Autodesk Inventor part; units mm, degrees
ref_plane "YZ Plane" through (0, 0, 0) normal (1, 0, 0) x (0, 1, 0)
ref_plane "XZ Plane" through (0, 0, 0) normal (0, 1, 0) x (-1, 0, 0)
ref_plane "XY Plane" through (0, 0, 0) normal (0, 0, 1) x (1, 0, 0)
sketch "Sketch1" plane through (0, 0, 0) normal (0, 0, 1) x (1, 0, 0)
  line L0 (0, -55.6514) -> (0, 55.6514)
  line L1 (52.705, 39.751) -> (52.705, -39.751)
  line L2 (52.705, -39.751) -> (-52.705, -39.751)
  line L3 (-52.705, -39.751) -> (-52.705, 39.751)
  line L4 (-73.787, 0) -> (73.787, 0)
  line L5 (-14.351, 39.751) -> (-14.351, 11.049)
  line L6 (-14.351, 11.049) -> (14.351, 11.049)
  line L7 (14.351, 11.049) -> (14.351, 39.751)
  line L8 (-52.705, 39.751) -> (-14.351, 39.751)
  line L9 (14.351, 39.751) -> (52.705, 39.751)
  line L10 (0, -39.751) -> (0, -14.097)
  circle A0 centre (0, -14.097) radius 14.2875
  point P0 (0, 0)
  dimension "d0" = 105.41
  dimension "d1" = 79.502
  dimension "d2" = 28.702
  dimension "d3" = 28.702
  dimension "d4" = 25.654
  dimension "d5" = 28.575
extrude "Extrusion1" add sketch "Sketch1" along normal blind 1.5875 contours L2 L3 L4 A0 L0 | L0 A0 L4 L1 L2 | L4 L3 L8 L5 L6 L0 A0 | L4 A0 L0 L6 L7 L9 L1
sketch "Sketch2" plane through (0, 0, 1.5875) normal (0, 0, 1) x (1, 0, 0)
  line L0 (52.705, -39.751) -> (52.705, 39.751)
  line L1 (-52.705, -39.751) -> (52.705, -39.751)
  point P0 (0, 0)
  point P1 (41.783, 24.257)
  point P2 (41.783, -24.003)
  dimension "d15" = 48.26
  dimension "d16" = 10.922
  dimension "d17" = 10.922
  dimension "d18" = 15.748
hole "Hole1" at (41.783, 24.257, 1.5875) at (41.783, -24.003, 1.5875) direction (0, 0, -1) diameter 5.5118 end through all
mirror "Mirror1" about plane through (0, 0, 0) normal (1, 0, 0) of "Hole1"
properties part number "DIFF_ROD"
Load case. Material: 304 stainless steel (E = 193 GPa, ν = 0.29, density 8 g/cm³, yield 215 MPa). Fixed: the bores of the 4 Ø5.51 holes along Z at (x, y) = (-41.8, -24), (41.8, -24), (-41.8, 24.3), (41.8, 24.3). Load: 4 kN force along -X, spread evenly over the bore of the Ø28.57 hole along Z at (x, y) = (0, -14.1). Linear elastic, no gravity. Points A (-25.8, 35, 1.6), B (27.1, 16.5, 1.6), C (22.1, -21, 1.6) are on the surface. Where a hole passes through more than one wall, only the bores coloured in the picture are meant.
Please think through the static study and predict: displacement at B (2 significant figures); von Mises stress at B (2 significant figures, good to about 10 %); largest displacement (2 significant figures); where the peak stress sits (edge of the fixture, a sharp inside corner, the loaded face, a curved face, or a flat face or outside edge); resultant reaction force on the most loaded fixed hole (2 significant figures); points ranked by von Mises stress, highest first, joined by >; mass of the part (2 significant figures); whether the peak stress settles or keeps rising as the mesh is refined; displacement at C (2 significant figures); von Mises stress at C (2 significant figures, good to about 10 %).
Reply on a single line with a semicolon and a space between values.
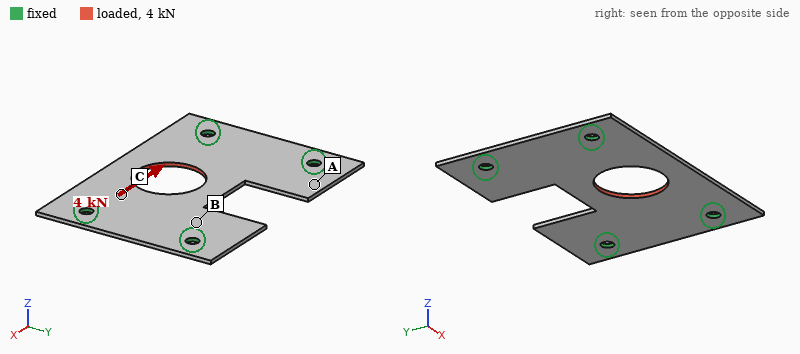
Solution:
1.9 µm; 19 MPa; 7.3 µm; edge of the fixture; 1.5 kN; C > B > A; 87 g; keeps rising; 4.3 µm; 35 MPa
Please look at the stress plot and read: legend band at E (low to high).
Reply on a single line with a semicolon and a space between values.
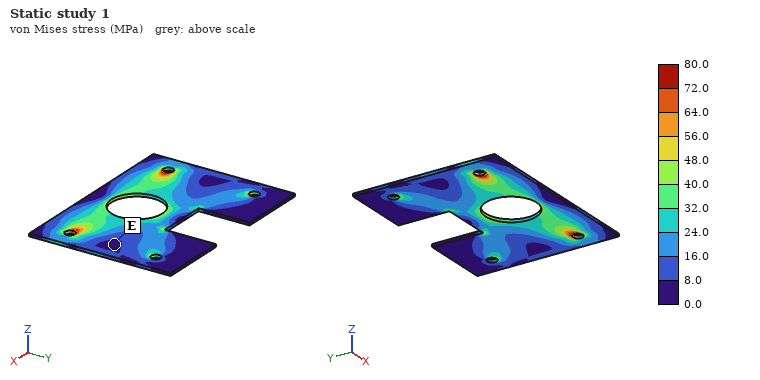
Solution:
0.0 to 8.0 MPa
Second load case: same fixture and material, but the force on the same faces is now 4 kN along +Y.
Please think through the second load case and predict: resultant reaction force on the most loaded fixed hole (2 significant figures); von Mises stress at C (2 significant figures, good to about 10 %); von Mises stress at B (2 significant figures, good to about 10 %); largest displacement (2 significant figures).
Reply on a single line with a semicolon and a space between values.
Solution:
1.3 kN; 42 MPa; 37 MPa; 19 µm
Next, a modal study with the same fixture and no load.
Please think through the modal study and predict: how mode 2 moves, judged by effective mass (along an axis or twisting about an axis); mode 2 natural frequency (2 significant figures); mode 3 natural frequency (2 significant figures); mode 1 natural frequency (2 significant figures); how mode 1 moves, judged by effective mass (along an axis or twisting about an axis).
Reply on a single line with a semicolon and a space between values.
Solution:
twisting about X; 1600 Hz; 2300 Hz; 1200 Hz; along Z
